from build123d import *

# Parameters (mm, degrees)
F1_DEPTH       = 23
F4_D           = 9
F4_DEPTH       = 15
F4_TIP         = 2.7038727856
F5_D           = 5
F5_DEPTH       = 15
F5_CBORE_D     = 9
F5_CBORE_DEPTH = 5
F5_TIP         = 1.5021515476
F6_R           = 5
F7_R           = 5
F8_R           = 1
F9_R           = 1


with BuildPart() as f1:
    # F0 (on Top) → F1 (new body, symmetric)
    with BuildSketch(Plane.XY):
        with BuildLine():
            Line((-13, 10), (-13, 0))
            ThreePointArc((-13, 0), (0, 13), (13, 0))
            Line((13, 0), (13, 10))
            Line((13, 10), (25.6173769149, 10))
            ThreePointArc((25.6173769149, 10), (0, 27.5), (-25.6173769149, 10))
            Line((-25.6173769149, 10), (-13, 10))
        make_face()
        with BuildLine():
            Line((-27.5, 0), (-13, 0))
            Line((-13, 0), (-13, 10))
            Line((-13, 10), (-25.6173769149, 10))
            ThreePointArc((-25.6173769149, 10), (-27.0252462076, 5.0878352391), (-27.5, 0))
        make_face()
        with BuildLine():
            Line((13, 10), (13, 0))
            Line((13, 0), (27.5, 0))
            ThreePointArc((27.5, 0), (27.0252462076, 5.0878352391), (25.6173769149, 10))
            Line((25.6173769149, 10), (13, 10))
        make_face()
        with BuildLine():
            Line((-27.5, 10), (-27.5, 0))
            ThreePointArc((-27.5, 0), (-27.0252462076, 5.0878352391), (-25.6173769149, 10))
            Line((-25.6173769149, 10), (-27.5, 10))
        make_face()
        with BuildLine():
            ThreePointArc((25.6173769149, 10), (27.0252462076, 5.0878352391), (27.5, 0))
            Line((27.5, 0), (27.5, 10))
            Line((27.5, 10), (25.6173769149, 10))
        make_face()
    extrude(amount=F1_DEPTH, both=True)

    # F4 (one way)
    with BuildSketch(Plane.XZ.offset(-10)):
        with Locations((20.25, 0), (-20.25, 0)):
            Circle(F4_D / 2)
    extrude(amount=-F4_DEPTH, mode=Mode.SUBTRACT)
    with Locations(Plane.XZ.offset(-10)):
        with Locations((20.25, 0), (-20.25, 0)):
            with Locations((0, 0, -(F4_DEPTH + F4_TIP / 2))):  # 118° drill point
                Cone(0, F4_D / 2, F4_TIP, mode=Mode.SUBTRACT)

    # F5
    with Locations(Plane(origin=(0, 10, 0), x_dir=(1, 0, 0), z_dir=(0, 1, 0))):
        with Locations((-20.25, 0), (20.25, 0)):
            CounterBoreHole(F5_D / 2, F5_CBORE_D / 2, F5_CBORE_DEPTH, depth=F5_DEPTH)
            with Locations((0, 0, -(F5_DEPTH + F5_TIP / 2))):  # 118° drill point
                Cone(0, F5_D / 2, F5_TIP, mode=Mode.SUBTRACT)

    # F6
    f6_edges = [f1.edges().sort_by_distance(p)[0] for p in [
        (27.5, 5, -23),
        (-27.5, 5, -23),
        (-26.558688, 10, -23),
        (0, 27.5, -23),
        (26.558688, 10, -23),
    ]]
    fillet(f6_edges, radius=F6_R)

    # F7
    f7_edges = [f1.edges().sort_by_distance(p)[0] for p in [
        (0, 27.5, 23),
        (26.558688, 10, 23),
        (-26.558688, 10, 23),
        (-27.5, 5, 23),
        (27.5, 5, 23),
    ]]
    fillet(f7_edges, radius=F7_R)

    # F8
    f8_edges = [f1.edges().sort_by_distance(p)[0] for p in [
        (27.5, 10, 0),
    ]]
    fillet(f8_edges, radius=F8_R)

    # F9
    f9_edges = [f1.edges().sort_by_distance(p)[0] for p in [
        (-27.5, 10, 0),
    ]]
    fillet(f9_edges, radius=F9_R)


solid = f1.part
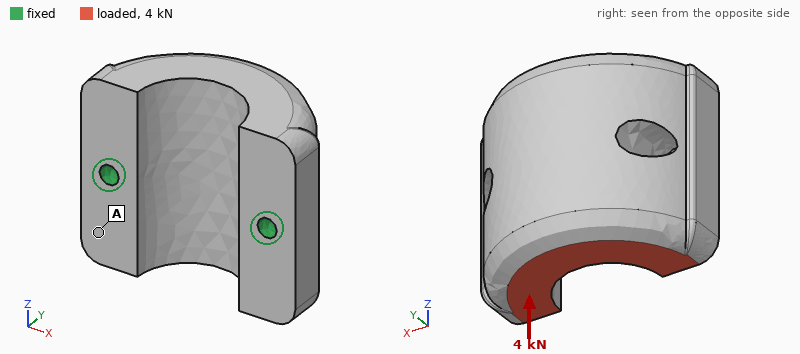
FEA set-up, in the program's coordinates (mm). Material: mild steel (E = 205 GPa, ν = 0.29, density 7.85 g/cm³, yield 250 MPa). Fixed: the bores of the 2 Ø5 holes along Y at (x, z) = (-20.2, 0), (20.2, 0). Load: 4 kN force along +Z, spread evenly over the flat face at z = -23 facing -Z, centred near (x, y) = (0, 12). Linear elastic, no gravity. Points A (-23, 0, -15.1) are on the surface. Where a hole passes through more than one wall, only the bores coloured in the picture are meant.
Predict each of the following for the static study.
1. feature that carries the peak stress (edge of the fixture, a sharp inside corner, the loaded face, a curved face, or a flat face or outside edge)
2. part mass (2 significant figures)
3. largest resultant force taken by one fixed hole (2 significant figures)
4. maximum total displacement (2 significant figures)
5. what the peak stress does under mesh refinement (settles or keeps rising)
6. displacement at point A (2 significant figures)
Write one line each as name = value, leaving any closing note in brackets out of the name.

feature that carries the peak stress = edge of the fixture
part mass = 320 g
largest resultant force taken by one fixed hole = 2.0 kN
maximum total displacement = 27 µm
what the peak stress does under mesh refinement = keeps rising
displacement at point A = 11 µm
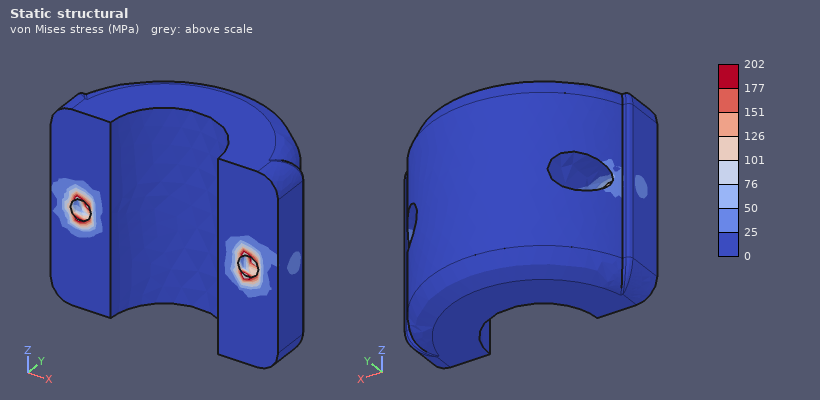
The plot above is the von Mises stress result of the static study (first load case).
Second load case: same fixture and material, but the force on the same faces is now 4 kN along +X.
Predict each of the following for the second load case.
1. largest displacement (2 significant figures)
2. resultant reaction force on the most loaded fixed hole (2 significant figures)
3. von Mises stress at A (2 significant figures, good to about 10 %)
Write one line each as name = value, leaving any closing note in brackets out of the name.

largest displacement = 10 µm
resultant reaction force on the most loaded fixed hole = 2.9 kN
von Mises stress at A = 14 MPa
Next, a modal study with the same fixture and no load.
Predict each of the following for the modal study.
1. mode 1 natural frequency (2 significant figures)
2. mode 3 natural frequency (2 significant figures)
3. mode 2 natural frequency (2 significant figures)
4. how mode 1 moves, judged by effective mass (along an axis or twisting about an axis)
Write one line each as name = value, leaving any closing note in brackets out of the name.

mode 1 natural frequency = 3200 Hz
mode 3 natural frequency = 12 kHz
mode 2 natural frequency = 11 kHz
how mode 1 moves, judged by effective mass = along Z
